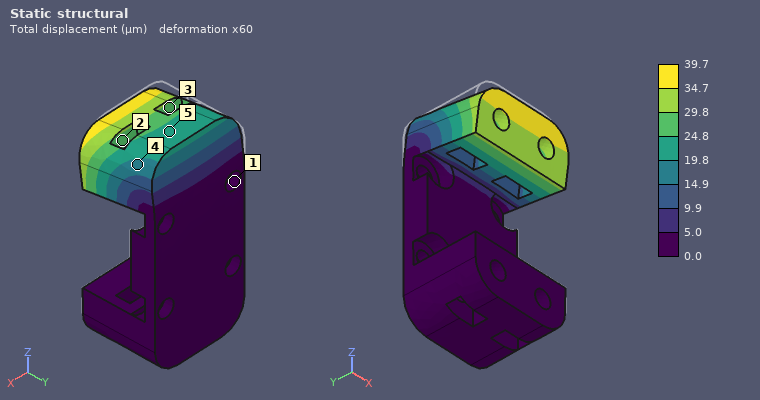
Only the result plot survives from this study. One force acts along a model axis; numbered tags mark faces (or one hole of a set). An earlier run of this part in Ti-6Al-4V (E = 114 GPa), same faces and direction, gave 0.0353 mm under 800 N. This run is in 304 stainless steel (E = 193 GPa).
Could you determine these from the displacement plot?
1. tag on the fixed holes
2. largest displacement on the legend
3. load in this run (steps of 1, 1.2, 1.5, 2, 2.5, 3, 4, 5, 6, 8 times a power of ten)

1
39.7 µm
1.5 kN
